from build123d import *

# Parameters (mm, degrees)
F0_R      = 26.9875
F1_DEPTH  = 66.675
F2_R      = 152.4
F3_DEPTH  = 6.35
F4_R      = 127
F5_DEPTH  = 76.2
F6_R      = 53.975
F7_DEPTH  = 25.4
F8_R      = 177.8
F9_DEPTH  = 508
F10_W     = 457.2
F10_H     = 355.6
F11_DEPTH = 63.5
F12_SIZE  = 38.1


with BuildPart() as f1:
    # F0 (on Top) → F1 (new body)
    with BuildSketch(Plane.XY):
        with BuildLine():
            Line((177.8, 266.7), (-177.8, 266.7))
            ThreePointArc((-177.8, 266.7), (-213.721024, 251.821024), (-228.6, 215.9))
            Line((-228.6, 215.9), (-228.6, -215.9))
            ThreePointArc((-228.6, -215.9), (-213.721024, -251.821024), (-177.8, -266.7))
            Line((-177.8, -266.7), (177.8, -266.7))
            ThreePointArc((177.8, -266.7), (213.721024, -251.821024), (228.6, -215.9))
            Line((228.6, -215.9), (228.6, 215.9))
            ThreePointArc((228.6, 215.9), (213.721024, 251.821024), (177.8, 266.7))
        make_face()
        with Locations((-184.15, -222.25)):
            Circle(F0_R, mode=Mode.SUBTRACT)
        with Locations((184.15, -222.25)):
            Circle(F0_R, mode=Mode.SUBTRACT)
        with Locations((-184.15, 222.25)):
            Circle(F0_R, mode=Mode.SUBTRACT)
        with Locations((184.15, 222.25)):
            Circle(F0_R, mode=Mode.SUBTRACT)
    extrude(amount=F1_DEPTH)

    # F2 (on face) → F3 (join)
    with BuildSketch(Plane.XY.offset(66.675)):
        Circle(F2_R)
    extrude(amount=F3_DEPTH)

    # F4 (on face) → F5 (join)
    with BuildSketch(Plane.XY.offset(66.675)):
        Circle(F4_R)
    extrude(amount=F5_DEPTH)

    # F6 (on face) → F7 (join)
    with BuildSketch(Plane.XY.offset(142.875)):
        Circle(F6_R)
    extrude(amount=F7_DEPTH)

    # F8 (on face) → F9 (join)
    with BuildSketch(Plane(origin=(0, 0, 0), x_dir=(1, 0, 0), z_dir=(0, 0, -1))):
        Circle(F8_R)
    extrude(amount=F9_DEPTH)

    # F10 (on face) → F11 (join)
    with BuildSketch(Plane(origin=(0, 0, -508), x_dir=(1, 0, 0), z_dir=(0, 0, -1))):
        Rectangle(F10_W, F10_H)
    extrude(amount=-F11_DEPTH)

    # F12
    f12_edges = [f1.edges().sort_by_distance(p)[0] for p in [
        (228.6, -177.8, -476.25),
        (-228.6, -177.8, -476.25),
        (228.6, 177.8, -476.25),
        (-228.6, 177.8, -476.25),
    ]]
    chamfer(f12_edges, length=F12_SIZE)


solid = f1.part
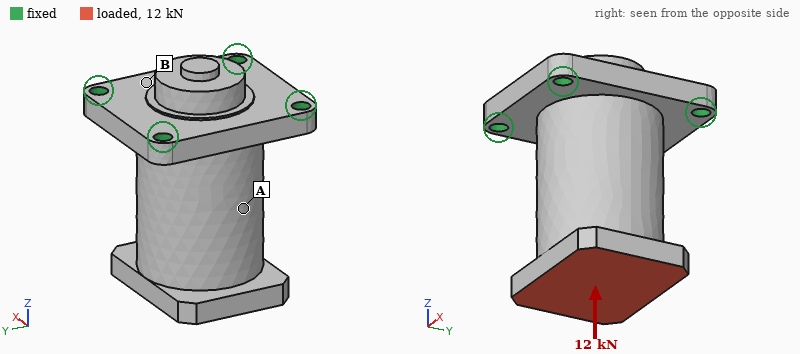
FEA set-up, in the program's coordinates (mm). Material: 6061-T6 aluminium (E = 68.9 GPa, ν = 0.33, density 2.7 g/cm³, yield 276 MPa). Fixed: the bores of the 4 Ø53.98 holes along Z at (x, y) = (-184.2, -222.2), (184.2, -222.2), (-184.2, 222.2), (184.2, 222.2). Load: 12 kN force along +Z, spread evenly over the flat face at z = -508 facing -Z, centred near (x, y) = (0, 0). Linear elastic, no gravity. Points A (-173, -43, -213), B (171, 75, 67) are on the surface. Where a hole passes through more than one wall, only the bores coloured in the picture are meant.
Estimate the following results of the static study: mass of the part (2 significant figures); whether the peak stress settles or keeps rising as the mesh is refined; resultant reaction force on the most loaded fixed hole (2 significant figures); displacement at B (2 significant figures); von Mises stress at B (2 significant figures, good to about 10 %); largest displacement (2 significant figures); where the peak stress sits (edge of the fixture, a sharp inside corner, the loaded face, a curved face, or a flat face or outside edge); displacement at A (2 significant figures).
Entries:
200 kg
keeps rising
3.1 kN
2.9 µm
0.49 MPa
5.3 µm
edge of the fixture
3.6 µm
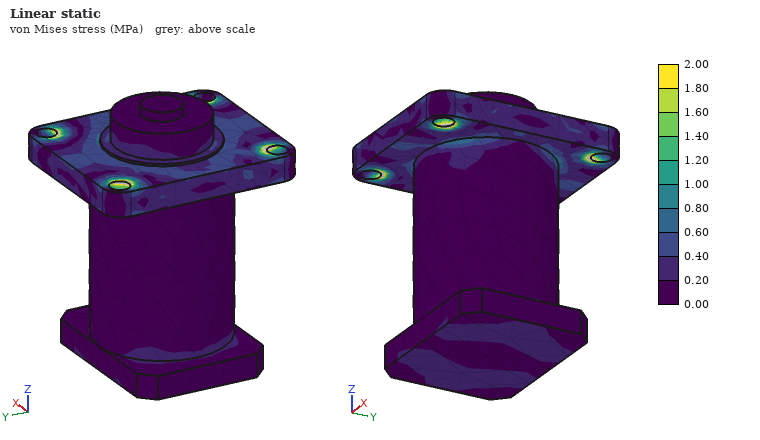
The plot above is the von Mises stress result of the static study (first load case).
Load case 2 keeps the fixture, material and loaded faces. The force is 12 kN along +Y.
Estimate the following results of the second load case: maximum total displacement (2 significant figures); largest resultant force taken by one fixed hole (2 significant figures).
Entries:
43 µm
9.2 kN
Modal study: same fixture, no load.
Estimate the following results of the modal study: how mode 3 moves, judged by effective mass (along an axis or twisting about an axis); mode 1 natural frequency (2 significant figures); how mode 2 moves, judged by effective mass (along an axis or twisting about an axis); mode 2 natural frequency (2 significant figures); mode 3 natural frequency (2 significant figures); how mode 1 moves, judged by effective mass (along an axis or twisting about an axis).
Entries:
along Z
310 Hz
along Y
360 Hz
690 Hz
along X
